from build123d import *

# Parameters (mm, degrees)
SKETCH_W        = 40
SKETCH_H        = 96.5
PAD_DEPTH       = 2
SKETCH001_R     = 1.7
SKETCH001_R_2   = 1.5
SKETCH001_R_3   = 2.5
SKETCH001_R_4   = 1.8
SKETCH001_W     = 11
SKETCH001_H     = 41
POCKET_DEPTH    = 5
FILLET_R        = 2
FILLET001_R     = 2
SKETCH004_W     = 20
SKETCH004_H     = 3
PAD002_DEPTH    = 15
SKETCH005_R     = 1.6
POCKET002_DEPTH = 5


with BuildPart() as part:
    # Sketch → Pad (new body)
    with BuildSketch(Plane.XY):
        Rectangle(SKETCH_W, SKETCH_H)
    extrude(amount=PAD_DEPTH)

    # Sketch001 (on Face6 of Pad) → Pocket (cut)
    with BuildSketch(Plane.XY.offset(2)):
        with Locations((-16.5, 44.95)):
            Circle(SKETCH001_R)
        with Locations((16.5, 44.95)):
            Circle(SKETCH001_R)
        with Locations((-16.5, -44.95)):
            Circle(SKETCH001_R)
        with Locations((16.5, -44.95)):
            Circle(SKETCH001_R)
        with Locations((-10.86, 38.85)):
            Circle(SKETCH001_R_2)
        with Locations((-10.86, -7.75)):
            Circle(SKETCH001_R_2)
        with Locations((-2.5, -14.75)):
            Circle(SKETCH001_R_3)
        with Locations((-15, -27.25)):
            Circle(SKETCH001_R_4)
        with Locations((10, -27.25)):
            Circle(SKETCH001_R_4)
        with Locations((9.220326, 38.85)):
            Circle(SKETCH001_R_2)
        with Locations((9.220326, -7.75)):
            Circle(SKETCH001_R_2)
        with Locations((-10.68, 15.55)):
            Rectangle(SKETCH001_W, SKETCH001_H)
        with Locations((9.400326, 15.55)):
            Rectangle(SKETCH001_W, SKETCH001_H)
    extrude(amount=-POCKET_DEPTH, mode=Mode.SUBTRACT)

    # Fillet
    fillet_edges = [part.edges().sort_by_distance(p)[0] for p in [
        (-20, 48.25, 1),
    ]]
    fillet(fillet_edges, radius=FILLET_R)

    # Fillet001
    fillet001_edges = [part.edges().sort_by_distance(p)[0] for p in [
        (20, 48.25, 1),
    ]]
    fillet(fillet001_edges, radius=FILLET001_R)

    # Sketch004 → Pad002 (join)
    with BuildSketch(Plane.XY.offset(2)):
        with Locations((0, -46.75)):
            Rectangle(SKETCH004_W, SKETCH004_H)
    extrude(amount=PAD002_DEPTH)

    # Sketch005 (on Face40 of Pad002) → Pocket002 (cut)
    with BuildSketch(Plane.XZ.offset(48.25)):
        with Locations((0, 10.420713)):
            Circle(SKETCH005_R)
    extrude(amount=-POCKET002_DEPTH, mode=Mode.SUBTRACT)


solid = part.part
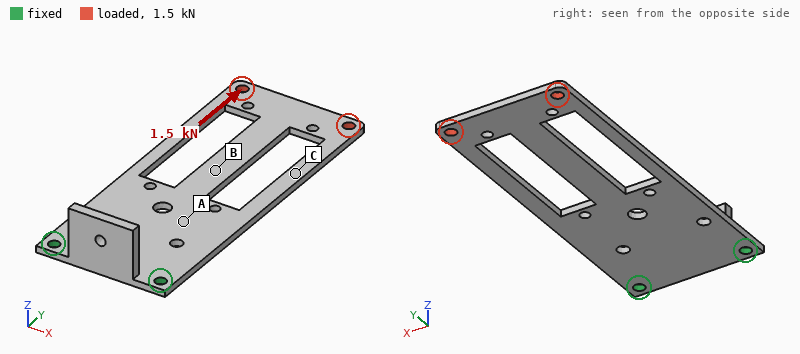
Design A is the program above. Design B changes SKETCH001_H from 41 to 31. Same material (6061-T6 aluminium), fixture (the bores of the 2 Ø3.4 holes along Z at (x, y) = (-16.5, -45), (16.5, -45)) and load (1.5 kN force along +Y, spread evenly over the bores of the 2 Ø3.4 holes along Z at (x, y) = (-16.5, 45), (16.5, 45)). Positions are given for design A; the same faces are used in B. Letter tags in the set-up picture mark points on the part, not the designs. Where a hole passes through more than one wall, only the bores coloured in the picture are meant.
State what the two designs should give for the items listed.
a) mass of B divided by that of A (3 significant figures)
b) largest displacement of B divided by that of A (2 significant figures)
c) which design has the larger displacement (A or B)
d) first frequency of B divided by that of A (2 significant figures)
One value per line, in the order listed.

1.07
0.88
A
0.96
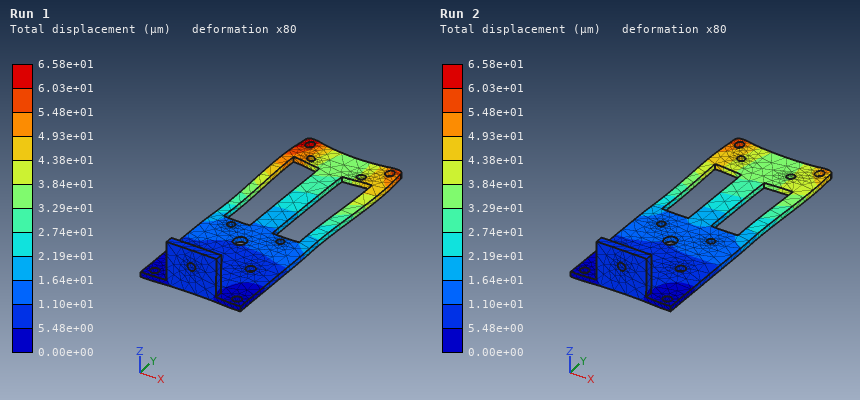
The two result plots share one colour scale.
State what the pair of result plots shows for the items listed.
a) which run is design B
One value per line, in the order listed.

Run 2
